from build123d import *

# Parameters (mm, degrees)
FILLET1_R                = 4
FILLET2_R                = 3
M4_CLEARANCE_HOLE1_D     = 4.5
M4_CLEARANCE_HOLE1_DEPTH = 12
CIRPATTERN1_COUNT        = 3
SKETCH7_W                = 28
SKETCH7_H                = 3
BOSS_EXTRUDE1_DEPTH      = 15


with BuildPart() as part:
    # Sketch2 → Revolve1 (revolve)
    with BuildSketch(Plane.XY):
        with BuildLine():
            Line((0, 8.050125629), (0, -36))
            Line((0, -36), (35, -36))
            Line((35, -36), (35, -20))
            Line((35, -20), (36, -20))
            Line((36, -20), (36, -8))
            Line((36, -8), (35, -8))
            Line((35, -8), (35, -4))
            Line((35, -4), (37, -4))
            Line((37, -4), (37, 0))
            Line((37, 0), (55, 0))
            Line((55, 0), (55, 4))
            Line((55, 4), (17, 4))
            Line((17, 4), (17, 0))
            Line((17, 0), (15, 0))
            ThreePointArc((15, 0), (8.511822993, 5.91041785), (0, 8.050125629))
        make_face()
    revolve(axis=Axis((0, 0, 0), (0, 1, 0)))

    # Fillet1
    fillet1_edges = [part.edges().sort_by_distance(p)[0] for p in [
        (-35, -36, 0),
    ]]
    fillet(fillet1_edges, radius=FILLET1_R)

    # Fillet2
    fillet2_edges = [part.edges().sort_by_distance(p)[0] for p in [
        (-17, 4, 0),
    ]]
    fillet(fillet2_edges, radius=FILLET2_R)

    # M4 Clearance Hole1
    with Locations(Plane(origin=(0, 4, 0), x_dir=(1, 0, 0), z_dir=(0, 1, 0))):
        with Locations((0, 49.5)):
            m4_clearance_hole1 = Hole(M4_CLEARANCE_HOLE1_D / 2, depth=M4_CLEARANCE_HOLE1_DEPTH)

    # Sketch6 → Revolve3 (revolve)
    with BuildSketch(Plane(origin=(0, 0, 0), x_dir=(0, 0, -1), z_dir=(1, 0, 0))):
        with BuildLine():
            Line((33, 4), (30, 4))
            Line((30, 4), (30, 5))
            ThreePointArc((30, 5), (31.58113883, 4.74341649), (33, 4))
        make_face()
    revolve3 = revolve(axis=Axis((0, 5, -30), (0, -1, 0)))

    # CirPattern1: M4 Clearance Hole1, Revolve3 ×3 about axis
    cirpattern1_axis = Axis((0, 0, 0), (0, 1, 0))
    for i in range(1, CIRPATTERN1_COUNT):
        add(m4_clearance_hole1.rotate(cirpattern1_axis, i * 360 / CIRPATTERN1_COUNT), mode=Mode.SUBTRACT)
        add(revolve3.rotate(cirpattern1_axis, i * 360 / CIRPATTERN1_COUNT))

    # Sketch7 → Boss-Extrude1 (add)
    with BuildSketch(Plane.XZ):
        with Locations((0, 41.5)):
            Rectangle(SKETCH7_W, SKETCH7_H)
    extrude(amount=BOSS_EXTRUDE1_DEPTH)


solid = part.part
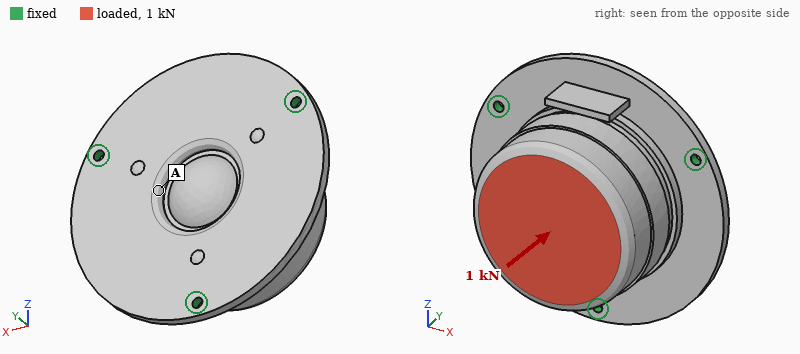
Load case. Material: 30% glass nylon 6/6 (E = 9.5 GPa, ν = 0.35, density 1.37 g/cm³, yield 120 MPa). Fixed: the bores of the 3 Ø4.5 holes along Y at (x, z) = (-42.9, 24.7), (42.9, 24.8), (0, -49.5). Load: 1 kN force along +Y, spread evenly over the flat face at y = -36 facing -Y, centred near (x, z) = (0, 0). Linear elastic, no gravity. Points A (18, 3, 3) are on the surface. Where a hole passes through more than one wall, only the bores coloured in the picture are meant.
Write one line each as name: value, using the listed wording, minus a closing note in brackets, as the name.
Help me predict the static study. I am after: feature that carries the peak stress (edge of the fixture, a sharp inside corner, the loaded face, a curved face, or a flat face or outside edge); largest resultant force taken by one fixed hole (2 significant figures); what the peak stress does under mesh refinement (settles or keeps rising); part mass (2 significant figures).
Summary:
feature that carries the peak stress: edge of the fixture
largest resultant force taken by one fixed hole: 370 N
what the peak stress does under mesh refinement: keeps rising
part mass: 250 g
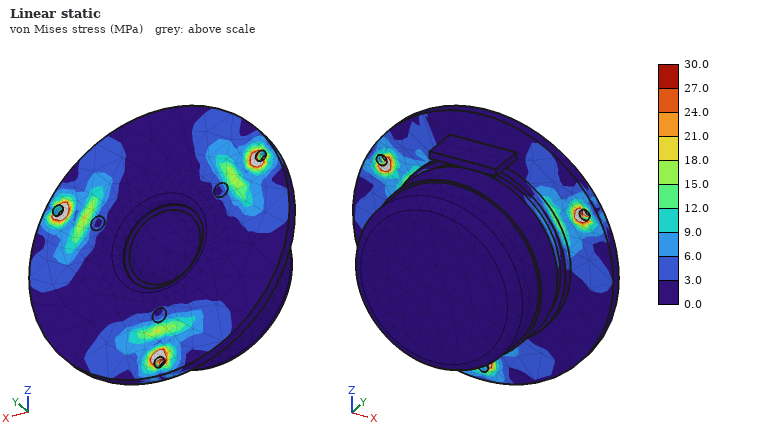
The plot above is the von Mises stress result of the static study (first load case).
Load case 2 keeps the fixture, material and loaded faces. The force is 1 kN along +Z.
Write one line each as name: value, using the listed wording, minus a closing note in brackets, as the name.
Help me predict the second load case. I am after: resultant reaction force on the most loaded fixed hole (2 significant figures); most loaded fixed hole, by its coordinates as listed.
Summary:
resultant reaction force on the most loaded fixed hole: 750 N
most loaded fixed hole, by its coordinates as listed: (0, -49.5)
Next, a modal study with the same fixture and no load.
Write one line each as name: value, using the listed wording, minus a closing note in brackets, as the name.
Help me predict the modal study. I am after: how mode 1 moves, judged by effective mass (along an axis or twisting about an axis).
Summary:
how mode 1 moves, judged by effective mass: along Y
